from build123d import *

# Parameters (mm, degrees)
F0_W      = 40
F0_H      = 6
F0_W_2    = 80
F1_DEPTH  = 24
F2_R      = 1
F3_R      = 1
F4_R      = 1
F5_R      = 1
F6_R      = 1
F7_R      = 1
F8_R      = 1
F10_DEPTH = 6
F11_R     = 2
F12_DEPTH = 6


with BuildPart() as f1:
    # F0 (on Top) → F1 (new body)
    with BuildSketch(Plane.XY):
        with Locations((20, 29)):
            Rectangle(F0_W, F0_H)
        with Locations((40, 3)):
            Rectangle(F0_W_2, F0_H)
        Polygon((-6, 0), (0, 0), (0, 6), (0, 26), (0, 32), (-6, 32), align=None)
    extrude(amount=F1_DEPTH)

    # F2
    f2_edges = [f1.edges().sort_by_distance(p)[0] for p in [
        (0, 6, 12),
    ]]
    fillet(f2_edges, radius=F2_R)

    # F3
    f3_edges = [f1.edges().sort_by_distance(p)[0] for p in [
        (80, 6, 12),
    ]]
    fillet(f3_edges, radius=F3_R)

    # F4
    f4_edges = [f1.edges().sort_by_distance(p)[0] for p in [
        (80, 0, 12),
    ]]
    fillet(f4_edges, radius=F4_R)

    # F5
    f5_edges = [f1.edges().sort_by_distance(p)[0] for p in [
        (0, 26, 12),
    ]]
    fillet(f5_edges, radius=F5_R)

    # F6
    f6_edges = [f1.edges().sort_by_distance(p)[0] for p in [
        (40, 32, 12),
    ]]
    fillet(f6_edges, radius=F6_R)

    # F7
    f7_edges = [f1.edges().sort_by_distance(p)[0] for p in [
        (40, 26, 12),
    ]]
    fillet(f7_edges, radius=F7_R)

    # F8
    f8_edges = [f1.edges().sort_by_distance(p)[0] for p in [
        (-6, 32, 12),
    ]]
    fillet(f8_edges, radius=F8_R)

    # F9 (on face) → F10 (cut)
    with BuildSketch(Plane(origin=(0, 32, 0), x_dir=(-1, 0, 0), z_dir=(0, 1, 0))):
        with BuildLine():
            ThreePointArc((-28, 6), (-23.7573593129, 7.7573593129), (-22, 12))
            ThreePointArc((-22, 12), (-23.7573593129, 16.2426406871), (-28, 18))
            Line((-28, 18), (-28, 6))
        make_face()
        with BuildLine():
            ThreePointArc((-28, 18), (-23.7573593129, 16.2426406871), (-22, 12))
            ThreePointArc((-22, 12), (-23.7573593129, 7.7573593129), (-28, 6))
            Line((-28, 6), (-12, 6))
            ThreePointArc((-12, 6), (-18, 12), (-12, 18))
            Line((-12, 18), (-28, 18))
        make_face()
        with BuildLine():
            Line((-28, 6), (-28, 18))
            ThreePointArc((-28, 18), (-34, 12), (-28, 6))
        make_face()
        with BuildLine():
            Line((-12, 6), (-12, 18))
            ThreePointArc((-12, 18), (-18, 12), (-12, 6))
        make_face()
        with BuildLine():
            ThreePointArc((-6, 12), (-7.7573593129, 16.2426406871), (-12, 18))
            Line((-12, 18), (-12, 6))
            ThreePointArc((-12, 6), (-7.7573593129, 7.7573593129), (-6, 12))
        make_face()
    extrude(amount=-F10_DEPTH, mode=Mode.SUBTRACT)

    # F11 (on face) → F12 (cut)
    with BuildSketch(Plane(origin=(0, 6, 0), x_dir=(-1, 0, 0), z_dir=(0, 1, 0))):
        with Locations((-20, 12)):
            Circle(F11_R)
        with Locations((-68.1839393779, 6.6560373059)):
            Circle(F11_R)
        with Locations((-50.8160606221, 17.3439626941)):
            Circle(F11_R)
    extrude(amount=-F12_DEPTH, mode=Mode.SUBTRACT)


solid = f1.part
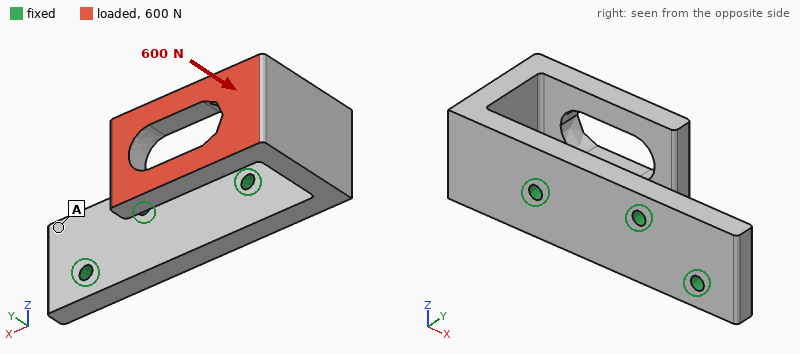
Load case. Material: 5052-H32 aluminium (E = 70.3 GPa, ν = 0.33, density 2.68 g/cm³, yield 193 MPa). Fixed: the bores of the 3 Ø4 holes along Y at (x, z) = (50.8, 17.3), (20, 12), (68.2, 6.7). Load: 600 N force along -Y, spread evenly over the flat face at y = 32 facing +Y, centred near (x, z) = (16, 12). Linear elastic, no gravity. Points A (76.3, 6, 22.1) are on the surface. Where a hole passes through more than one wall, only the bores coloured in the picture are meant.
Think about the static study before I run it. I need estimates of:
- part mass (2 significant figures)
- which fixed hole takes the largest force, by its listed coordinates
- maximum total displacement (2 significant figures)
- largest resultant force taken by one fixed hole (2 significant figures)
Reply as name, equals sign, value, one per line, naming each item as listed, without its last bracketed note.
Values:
part mass = 53 g
which fixed hole takes the largest force, by its listed coordinates = (20, 12)
maximum total displacement = 0.72 mm
largest resultant force taken by one fixed hole = 620 N
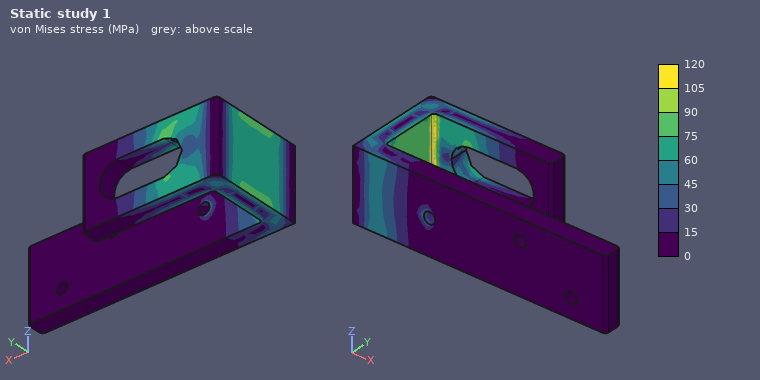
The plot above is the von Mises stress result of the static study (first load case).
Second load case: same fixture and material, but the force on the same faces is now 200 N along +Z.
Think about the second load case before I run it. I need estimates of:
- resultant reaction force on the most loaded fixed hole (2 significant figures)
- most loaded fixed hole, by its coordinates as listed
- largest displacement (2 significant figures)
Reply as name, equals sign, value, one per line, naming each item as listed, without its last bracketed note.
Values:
resultant reaction force on the most loaded fixed hole = 220 N
most loaded fixed hole, by its coordinates as listed = (20, 12)
largest displacement = 0.21 mm
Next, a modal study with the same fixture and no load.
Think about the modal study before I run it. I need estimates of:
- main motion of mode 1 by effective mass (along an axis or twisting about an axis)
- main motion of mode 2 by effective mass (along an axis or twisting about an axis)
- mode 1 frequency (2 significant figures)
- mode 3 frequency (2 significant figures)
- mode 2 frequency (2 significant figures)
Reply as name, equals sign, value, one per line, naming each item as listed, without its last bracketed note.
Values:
main motion of mode 1 by effective mass = along X
main motion of mode 2 by effective mass = along Z
mode 1 frequency = 1200 Hz
mode 3 frequency = 2400 Hz
mode 2 frequency = 1600 Hz
